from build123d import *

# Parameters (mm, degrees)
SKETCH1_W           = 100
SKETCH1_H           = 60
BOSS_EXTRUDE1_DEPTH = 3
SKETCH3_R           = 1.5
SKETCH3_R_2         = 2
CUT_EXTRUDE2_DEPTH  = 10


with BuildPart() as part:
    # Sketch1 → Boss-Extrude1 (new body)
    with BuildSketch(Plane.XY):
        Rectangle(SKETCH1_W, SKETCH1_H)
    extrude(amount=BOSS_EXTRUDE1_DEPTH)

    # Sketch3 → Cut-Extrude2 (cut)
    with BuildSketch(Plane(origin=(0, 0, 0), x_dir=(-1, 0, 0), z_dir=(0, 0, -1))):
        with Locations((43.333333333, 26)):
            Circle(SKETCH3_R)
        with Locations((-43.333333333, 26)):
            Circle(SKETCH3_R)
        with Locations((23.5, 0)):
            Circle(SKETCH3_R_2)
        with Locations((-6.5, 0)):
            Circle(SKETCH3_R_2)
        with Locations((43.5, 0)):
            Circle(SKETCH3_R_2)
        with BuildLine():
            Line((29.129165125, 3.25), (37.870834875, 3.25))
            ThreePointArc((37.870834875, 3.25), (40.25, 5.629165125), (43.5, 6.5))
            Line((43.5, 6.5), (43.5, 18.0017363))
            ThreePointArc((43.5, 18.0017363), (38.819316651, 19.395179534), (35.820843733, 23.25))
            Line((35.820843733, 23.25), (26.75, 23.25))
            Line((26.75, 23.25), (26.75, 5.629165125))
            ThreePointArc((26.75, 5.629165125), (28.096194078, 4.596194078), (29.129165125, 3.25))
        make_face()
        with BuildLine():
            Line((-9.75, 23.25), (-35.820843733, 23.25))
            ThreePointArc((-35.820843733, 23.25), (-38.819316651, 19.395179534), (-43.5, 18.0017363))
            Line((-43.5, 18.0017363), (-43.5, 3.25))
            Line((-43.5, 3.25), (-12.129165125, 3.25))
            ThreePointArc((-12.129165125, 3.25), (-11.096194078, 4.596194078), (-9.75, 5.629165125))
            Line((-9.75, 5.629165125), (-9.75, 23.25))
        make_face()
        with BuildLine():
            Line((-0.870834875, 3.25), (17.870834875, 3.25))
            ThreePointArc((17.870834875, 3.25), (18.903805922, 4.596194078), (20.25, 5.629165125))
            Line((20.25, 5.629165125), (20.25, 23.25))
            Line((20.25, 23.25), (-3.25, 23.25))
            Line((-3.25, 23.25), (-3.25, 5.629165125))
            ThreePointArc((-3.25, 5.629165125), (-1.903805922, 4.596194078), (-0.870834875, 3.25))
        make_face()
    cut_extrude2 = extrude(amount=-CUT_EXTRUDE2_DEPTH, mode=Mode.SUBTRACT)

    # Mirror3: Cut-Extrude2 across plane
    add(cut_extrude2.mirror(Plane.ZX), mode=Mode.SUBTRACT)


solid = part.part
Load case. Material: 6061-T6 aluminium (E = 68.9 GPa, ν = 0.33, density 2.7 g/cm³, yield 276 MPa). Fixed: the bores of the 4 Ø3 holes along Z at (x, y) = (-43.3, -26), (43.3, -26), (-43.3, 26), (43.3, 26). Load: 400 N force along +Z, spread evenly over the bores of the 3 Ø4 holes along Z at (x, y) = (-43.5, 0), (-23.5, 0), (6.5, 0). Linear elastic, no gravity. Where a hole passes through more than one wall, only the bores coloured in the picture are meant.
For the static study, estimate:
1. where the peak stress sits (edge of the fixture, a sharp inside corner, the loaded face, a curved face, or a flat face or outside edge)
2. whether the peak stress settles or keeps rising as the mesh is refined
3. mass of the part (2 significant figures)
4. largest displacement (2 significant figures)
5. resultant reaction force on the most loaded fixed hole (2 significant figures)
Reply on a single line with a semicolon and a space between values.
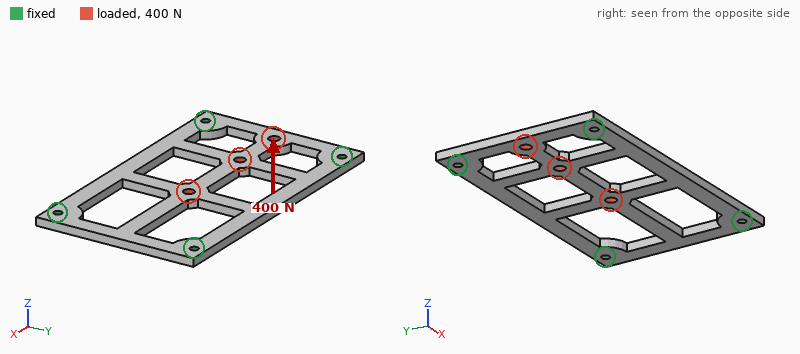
edge of the fixture; keeps rising; 25 g; 0.34 mm; 150 N
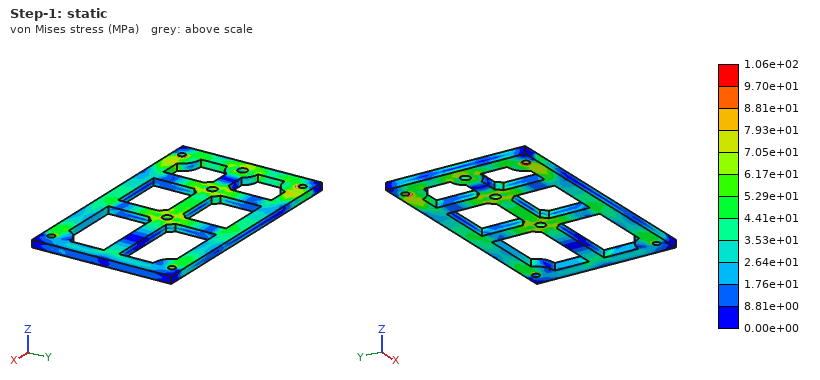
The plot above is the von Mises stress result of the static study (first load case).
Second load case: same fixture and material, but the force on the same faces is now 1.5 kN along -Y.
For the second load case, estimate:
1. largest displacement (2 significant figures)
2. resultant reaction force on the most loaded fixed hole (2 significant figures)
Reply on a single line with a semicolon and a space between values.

80 µm; 640 N
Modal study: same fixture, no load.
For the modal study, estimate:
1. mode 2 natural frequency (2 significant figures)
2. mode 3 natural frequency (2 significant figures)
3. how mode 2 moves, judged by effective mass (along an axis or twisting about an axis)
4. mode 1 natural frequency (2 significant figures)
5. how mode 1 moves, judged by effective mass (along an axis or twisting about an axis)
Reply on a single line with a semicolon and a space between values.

2500 Hz; 3800 Hz; twisting about X; 1600 Hz; along Z
